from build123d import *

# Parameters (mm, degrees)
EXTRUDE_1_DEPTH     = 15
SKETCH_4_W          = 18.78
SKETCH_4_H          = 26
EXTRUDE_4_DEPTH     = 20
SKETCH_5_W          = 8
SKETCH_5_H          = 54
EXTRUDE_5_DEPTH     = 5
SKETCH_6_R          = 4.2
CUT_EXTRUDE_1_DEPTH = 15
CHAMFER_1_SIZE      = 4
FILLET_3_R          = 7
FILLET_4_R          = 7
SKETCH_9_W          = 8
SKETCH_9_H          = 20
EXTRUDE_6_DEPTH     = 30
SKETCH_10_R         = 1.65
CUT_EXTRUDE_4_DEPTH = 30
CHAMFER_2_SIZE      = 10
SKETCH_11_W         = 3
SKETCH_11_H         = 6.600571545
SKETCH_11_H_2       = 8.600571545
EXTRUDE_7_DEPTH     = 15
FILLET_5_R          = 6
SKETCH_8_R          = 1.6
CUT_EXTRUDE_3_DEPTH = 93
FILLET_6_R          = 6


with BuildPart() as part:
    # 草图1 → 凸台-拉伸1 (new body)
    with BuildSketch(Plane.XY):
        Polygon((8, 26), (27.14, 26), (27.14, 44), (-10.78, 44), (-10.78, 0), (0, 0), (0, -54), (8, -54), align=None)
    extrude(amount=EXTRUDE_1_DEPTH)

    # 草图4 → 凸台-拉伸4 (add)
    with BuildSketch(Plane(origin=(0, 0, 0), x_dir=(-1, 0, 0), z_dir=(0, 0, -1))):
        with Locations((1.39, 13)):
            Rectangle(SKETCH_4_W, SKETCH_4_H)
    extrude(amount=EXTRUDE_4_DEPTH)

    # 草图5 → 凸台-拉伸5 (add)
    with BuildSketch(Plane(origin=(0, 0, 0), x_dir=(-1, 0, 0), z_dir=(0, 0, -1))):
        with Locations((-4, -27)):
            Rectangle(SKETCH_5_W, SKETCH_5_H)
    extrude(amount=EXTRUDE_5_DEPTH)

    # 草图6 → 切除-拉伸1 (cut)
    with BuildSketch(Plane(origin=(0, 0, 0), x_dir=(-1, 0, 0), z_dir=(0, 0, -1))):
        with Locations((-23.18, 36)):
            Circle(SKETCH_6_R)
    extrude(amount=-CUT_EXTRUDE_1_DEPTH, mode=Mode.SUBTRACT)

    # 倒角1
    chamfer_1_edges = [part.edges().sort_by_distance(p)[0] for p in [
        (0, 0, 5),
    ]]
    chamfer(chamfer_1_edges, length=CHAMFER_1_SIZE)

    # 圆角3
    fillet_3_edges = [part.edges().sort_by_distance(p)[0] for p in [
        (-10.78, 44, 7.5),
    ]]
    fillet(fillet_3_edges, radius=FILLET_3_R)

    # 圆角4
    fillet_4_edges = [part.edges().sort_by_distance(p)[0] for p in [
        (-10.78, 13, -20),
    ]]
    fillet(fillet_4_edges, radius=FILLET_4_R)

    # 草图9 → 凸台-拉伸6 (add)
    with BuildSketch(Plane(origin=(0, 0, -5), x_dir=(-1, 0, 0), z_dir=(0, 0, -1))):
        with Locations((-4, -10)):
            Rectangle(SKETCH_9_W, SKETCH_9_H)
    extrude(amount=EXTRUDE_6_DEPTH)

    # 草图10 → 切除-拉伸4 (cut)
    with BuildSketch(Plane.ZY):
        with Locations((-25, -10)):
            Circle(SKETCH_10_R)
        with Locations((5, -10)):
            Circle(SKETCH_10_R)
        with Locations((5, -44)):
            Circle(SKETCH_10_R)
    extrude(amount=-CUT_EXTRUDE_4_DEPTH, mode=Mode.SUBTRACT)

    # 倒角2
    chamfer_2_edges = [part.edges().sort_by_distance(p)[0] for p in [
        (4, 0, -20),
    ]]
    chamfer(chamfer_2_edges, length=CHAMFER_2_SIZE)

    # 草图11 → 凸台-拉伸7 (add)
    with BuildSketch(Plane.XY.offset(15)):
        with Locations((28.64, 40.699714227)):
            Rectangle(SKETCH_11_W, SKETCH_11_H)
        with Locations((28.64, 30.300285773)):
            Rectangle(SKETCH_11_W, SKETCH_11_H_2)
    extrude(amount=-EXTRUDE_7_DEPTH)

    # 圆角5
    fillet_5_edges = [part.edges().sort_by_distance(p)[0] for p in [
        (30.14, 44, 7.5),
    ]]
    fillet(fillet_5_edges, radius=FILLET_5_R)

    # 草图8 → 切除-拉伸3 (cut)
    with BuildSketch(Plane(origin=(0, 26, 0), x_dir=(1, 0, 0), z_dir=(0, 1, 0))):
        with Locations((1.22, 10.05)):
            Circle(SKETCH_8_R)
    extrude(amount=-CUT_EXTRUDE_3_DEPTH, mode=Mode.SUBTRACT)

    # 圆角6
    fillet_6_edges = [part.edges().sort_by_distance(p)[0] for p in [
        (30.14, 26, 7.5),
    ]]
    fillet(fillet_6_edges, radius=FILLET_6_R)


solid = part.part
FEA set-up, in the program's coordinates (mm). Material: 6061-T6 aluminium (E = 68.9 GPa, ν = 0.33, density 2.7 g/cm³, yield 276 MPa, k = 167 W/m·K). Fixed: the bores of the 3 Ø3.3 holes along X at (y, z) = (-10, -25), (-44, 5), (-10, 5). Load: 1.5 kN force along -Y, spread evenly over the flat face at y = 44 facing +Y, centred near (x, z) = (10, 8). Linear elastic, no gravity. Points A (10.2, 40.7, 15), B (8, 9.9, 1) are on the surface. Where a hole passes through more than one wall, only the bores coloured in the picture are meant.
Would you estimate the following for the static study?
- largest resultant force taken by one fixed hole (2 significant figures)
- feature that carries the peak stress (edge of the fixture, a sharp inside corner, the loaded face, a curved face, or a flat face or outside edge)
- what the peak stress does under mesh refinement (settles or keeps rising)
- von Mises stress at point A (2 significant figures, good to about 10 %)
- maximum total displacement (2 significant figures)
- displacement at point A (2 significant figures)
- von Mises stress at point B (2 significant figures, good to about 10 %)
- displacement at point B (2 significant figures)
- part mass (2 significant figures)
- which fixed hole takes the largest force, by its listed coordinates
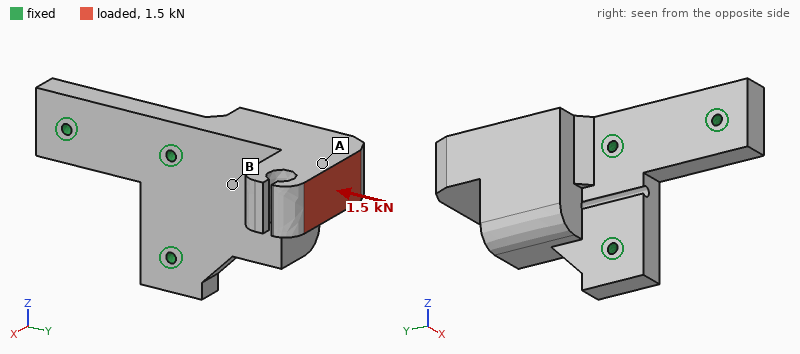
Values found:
1.4 kN
edge of the fixture
keeps rising
6.2 MPa
94 µm
71 µm
16 MPa
19 µm
110 g
(-10, 5)
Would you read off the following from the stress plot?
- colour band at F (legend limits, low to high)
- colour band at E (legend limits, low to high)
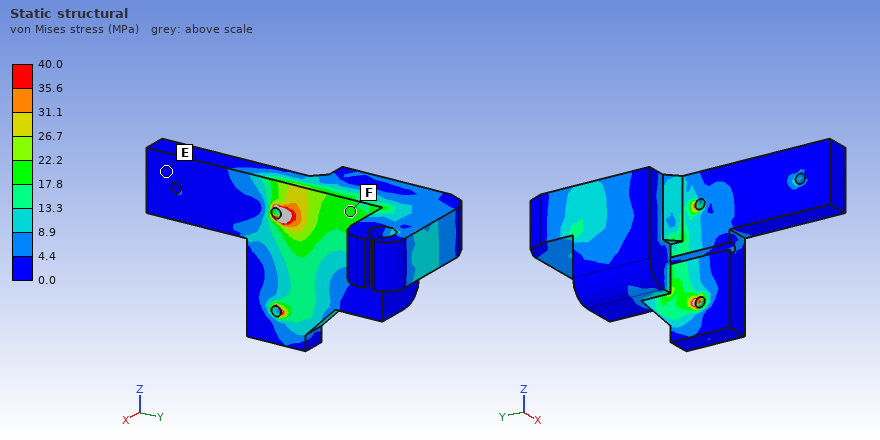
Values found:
17.8 to 22.2 MPa
0.0 to 4.4 MPa
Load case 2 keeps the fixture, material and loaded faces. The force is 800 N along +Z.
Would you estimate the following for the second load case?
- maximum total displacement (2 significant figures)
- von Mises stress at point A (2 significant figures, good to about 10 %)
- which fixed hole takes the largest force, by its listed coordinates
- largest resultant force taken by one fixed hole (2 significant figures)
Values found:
55 µm
6.0 MPa
(-10, -25)
1.5 kN
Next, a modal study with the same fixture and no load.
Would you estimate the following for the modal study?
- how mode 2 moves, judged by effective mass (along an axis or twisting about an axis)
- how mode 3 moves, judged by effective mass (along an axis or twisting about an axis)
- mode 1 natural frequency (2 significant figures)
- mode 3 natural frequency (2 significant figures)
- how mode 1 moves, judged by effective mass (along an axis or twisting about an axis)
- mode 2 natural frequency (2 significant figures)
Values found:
along Z
along Z
1700 Hz
7700 Hz
along X
5200 Hz
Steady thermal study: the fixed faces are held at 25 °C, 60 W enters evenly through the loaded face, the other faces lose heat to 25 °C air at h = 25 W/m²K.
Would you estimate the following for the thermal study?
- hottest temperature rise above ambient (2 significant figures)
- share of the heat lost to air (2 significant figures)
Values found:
61 K
9.2 %
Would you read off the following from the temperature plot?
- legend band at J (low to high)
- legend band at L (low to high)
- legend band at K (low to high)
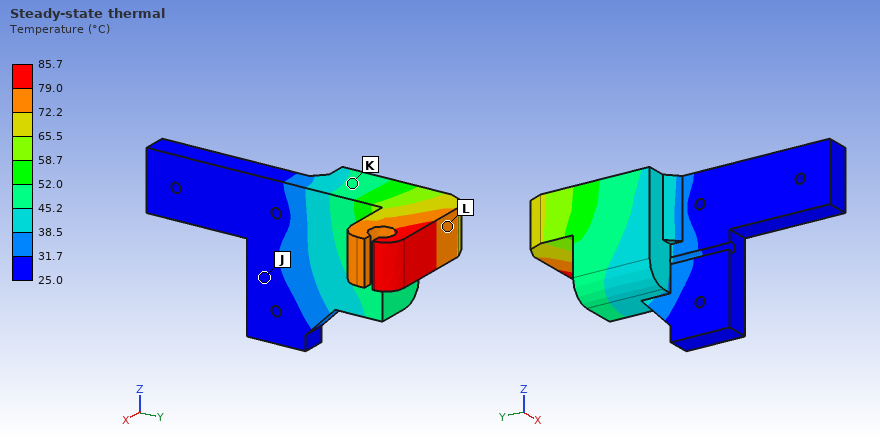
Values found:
25.0 to 31.7 °C
72.2 to 79.0 °C
45.2 to 52.0 °C
